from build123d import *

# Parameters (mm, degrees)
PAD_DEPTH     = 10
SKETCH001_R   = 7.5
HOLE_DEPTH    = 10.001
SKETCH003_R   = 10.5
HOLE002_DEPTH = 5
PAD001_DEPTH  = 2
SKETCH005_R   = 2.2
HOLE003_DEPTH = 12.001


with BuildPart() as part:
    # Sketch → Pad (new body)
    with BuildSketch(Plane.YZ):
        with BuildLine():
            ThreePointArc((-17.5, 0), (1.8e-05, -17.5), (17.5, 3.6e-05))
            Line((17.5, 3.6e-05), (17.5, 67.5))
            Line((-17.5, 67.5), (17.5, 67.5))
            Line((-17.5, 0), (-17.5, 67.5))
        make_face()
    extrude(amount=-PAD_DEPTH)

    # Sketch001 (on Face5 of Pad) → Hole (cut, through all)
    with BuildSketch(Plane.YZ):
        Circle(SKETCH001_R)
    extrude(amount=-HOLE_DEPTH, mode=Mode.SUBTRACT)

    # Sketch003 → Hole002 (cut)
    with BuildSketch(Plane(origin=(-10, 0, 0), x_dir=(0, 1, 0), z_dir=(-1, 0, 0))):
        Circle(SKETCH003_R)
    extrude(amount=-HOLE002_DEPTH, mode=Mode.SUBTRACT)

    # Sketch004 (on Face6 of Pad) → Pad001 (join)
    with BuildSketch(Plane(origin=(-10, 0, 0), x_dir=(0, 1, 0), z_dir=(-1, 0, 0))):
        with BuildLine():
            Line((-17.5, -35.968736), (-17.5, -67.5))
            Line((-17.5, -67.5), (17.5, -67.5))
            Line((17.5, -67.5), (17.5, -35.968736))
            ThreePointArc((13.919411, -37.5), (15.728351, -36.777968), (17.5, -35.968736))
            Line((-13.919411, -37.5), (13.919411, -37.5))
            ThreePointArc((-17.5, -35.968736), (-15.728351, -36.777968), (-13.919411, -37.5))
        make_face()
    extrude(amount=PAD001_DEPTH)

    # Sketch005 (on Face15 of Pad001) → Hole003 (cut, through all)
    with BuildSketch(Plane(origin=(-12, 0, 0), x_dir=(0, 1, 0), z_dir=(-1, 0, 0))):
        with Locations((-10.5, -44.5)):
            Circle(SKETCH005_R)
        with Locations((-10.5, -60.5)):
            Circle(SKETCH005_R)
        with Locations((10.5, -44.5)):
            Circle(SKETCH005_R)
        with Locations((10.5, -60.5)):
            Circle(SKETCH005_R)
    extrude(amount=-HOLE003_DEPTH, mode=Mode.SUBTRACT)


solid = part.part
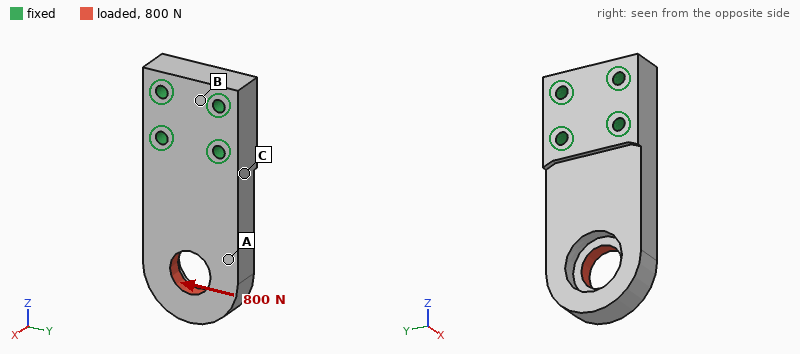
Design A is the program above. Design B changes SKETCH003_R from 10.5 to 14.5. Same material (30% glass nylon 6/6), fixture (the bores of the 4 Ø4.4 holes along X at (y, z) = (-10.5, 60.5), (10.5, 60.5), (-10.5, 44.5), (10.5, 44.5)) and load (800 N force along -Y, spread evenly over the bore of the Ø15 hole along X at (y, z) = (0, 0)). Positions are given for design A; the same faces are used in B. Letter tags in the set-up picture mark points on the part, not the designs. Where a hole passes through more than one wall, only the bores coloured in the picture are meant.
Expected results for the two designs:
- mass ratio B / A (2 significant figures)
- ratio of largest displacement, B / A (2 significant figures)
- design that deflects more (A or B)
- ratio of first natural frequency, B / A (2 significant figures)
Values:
0.94
1.1
B
1.1
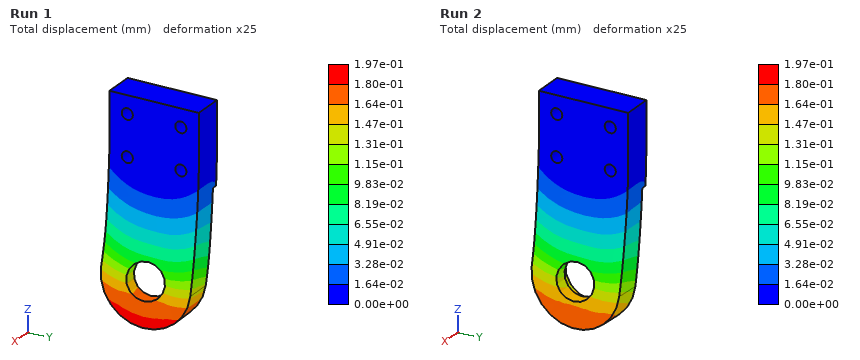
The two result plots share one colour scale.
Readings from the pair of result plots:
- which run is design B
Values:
Run 1
